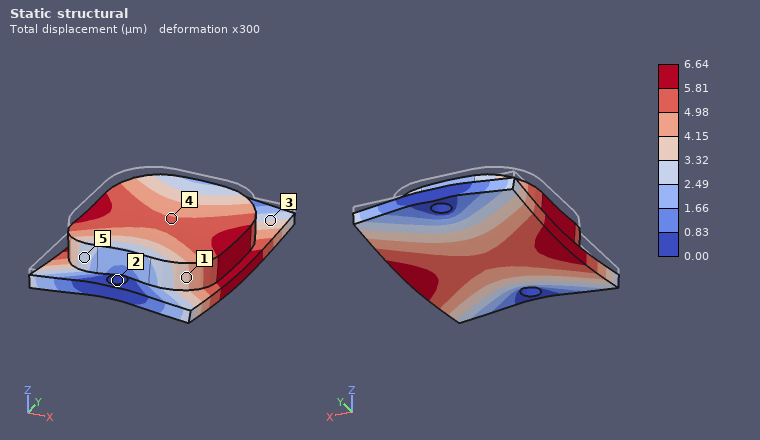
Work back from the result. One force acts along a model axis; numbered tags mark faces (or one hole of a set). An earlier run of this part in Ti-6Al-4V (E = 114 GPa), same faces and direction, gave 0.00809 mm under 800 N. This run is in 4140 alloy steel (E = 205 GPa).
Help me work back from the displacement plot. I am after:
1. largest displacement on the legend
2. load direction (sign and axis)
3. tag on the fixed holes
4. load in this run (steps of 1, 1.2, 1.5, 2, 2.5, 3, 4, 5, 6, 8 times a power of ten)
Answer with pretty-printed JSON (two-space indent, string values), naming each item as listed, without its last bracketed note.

{
  "largest displacement on the legend": "6.64 µm",
  "load direction": "-Z",
  "tag on the fixed holes": "2",
  "load in this run": "1.2 kN"
}
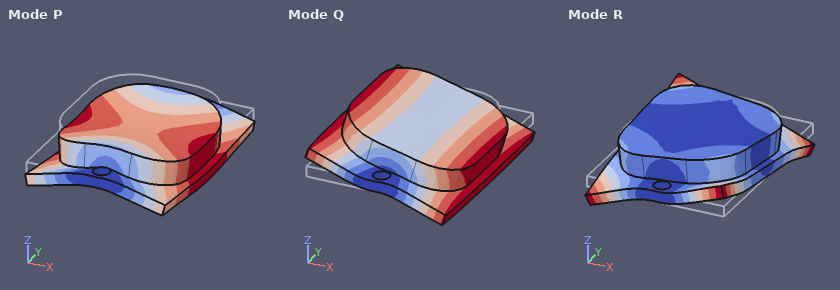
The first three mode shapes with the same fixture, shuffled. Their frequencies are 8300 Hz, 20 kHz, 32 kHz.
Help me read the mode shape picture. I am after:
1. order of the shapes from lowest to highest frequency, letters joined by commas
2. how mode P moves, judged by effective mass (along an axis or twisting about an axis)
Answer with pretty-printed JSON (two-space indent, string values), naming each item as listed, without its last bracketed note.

{
  "order of the shapes from lowest to highest frequency, letters joined by commas": "Q, P, R",
  "how mode P moves, judged by effective mass": "along Z"
}
